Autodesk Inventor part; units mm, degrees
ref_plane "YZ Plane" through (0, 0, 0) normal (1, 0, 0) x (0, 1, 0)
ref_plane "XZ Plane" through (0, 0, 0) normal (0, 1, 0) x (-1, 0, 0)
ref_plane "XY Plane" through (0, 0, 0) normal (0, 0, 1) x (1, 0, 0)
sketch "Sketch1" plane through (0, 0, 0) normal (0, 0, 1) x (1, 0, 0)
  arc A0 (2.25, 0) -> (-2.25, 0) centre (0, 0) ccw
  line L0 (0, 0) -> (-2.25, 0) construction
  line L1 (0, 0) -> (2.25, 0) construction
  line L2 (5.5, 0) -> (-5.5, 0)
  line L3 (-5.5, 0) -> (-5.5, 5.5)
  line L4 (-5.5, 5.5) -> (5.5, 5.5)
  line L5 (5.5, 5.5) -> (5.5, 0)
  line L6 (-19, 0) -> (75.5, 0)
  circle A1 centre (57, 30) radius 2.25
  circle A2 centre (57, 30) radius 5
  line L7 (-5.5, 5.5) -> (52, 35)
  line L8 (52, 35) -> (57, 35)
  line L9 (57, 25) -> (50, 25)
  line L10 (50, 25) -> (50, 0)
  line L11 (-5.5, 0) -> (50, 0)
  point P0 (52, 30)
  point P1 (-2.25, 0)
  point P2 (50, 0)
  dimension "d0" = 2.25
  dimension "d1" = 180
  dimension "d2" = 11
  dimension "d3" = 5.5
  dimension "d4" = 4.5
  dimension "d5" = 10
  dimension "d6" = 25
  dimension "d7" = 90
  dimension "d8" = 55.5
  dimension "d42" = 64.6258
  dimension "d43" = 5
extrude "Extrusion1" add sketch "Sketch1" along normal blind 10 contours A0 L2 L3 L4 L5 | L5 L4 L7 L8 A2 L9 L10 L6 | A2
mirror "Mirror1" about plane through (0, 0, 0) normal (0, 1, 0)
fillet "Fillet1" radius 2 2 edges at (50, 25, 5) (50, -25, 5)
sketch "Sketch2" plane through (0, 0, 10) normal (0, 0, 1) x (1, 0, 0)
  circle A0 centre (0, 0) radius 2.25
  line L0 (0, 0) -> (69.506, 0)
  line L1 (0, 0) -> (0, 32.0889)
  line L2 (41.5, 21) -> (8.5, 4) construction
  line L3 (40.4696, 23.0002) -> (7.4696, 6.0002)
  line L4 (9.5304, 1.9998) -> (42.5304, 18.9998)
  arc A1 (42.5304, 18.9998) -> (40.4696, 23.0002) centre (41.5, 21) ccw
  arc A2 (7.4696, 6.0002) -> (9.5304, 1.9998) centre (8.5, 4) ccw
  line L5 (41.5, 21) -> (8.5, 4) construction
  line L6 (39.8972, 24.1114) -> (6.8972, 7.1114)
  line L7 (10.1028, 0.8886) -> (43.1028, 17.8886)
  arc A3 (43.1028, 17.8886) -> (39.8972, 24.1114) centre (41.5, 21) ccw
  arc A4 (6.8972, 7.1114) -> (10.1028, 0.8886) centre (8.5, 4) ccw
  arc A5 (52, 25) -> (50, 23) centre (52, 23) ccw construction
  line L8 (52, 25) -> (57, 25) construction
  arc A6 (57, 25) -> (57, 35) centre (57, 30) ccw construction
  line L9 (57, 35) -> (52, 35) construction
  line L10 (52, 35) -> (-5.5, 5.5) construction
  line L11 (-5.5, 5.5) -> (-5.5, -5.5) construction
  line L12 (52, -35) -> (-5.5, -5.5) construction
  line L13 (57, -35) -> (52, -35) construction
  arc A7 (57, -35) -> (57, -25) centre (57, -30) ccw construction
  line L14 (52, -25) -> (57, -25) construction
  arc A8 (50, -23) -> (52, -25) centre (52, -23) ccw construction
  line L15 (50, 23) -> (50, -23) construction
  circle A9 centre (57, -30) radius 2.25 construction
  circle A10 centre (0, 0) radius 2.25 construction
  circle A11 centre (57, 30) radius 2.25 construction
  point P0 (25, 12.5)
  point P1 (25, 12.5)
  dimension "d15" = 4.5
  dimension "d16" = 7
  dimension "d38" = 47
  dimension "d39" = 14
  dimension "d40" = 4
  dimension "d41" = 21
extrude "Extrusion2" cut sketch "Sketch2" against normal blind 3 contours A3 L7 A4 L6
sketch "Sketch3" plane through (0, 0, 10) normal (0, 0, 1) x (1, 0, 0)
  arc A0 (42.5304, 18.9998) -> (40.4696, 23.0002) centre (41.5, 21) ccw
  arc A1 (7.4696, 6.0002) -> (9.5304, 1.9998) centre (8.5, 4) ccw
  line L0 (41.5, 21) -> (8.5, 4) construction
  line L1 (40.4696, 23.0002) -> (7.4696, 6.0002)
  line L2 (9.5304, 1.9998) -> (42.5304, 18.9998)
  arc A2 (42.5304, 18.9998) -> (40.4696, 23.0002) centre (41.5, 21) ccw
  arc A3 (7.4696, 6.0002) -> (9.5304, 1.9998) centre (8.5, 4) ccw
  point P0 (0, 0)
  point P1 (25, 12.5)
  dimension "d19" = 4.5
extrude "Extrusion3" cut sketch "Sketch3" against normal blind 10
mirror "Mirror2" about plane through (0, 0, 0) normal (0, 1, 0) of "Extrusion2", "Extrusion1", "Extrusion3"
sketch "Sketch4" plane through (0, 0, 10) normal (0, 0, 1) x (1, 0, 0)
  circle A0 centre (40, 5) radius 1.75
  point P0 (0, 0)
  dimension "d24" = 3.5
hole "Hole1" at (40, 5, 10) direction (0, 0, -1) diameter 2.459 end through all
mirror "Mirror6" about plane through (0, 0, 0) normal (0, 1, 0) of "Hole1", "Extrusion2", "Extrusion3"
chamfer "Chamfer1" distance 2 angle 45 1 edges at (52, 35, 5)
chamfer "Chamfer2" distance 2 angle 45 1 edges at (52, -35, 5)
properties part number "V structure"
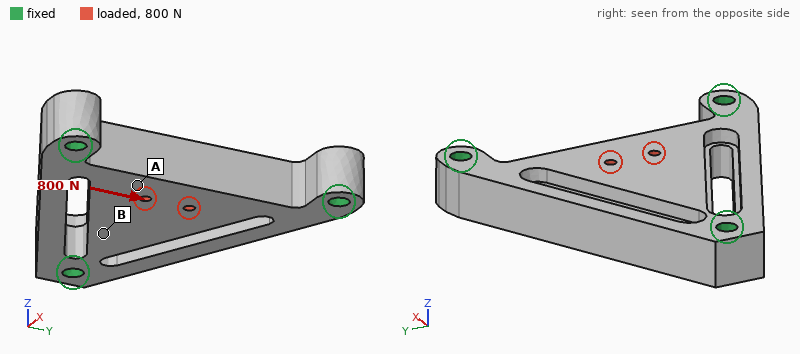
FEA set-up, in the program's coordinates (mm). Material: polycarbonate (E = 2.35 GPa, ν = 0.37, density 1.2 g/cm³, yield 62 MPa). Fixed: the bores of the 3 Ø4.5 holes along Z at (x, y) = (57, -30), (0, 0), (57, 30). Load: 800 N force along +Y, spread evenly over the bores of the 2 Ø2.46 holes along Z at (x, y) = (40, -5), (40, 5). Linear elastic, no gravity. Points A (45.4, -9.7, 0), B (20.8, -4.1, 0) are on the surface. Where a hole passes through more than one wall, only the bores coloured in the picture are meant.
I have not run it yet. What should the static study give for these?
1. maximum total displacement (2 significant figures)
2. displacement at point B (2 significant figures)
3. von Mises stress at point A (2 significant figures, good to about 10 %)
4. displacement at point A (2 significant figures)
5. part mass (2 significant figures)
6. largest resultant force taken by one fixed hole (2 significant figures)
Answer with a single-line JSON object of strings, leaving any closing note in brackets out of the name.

{"maximum total displacement": "0.12 mm", "displacement at point B": "0.064 mm", "von Mises stress at point A": "3.9 MPa", "displacement at point A": "0.11 mm", "part mass": "23 g", "largest resultant force taken by one fixed hole": "350 N"}
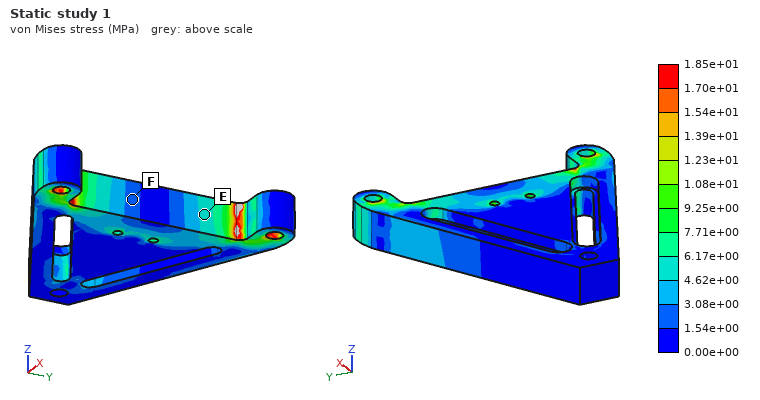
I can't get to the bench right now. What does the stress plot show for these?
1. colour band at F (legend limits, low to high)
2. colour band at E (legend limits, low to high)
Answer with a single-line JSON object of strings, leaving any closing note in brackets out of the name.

{"colour band at F": "1.54e+00 to 3.08e+00 MPa", "colour band at E": "4.62e+00 to 6.17e+00 MPa"}
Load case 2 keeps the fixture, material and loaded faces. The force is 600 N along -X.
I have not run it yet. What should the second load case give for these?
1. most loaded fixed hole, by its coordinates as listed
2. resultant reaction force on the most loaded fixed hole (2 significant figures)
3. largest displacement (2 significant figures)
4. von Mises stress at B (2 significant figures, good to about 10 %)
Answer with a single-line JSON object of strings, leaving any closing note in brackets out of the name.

{"most loaded fixed hole, by its coordinates as listed": "(0, 0)", "resultant reaction force on the most loaded fixed hole": "370 N", "largest displacement": "83 µm", "von Mises stress at B": "3.0 MPa"}
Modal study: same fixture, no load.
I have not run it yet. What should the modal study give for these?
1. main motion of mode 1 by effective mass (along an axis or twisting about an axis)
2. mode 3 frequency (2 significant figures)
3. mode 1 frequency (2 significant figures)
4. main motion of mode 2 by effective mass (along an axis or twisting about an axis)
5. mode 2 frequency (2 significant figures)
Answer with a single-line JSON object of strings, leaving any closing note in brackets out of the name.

{"main motion of mode 1 by effective mass": "along Z", "mode 3 frequency": "3100 Hz", "mode 1 frequency": "2100 Hz", "main motion of mode 2 by effective mass": "along Y", "mode 2 frequency": "2800 Hz"}
